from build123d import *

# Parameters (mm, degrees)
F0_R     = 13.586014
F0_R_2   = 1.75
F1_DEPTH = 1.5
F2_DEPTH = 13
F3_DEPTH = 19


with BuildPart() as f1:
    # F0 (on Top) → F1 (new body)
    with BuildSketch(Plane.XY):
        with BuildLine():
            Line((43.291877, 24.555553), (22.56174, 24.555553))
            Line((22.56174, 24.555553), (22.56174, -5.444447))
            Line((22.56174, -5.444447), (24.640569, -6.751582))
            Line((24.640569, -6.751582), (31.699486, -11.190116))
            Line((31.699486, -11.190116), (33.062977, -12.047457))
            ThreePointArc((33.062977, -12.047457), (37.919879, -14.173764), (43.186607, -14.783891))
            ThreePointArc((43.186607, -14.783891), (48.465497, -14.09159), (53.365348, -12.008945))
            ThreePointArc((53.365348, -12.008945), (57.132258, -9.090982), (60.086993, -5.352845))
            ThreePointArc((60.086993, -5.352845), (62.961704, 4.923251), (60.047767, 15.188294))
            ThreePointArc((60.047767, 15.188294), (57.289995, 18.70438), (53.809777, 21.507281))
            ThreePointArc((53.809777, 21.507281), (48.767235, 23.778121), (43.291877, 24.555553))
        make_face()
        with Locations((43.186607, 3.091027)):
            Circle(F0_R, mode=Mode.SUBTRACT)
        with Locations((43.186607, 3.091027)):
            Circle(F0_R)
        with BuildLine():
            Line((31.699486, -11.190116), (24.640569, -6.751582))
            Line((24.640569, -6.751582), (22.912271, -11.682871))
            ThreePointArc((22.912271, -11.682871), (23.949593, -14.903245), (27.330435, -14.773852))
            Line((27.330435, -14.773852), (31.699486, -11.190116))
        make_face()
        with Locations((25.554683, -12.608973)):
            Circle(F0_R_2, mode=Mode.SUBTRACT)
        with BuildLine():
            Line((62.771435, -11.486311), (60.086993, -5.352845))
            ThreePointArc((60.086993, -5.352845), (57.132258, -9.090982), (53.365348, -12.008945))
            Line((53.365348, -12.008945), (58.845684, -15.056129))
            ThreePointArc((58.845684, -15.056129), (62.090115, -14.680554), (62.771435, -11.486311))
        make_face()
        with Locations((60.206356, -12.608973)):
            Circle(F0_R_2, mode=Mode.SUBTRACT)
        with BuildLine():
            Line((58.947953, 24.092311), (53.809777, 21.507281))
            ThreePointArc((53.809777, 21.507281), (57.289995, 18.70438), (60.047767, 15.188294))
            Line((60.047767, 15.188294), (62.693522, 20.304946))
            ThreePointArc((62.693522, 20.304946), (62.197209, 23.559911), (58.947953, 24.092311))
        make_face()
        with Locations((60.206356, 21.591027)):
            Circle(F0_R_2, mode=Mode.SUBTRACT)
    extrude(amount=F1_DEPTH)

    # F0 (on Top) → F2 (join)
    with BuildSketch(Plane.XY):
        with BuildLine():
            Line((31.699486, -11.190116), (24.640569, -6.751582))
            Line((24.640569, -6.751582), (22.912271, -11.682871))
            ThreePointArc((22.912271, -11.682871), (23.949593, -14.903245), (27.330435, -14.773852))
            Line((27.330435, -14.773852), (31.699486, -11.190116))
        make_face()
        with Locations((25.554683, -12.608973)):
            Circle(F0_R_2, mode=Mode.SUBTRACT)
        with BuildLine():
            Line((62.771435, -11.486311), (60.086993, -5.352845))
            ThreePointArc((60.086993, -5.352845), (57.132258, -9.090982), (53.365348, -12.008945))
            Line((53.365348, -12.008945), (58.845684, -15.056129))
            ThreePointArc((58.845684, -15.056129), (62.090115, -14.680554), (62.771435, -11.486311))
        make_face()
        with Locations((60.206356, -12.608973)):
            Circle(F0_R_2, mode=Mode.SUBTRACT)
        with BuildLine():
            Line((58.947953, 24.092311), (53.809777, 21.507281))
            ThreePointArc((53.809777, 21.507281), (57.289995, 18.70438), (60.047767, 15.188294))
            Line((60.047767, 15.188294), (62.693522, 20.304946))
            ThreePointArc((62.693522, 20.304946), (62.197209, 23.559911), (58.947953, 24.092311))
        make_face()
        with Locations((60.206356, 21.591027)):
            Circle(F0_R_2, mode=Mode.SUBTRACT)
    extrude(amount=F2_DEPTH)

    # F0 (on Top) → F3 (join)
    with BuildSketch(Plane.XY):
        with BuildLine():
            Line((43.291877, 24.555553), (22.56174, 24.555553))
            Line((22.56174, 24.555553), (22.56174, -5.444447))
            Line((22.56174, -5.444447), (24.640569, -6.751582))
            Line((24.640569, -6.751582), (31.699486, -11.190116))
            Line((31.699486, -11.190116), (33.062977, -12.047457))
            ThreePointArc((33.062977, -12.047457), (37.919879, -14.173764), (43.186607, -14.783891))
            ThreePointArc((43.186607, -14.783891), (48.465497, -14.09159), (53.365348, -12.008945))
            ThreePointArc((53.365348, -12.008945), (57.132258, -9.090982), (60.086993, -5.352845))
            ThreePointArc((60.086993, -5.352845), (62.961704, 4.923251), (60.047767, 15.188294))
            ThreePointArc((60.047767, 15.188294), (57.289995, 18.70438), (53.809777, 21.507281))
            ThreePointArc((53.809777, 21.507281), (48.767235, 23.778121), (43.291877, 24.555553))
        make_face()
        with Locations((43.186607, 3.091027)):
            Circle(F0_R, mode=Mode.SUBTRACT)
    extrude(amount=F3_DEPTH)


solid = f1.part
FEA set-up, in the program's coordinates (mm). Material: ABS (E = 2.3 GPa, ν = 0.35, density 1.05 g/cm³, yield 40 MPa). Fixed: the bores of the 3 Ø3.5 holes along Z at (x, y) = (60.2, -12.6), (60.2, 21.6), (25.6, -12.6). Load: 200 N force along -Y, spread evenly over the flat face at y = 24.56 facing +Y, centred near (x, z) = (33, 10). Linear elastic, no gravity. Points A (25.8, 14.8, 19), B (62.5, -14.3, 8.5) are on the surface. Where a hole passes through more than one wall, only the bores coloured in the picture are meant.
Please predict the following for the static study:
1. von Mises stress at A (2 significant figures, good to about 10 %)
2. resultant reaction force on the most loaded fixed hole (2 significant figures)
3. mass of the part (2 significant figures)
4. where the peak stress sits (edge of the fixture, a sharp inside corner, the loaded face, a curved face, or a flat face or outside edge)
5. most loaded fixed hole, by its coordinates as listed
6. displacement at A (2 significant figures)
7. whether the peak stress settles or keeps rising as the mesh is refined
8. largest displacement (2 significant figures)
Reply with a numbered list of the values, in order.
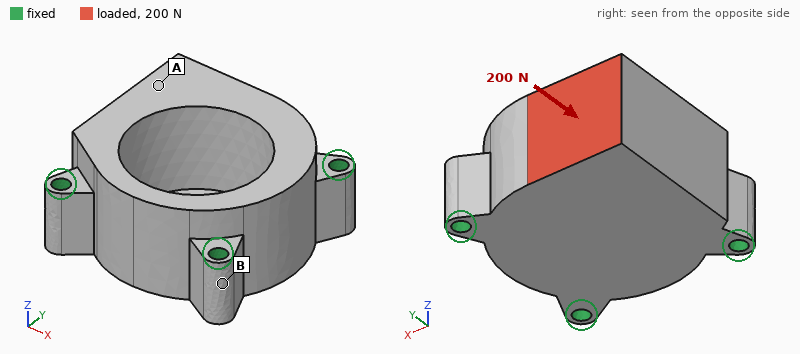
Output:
1. 0.91 MPa
2. 150 N
3. 18 g
4. edge of the fixture
5. (25.6, -12.6)
6. 26 µm
7. keeps rising
8. 34 µm
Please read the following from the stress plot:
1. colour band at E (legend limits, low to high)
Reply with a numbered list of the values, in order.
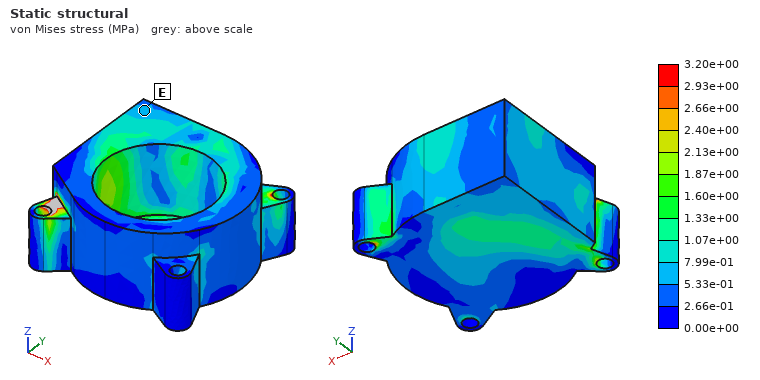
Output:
1. 5.33e-01 to 7.99e-01 MPa
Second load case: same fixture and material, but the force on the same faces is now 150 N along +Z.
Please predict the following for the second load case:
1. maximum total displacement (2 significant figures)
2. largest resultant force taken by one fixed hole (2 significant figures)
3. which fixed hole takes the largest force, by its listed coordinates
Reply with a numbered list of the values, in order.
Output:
1. 0.18 mm
2. 130 N
3. (60.2, 21.6)
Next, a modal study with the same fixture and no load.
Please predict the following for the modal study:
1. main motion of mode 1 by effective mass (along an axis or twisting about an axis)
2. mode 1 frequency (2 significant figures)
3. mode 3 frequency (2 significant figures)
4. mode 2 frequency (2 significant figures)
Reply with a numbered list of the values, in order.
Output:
1. along Z
2. 2400 Hz
3. 5700 Hz
4. 5200 Hz
